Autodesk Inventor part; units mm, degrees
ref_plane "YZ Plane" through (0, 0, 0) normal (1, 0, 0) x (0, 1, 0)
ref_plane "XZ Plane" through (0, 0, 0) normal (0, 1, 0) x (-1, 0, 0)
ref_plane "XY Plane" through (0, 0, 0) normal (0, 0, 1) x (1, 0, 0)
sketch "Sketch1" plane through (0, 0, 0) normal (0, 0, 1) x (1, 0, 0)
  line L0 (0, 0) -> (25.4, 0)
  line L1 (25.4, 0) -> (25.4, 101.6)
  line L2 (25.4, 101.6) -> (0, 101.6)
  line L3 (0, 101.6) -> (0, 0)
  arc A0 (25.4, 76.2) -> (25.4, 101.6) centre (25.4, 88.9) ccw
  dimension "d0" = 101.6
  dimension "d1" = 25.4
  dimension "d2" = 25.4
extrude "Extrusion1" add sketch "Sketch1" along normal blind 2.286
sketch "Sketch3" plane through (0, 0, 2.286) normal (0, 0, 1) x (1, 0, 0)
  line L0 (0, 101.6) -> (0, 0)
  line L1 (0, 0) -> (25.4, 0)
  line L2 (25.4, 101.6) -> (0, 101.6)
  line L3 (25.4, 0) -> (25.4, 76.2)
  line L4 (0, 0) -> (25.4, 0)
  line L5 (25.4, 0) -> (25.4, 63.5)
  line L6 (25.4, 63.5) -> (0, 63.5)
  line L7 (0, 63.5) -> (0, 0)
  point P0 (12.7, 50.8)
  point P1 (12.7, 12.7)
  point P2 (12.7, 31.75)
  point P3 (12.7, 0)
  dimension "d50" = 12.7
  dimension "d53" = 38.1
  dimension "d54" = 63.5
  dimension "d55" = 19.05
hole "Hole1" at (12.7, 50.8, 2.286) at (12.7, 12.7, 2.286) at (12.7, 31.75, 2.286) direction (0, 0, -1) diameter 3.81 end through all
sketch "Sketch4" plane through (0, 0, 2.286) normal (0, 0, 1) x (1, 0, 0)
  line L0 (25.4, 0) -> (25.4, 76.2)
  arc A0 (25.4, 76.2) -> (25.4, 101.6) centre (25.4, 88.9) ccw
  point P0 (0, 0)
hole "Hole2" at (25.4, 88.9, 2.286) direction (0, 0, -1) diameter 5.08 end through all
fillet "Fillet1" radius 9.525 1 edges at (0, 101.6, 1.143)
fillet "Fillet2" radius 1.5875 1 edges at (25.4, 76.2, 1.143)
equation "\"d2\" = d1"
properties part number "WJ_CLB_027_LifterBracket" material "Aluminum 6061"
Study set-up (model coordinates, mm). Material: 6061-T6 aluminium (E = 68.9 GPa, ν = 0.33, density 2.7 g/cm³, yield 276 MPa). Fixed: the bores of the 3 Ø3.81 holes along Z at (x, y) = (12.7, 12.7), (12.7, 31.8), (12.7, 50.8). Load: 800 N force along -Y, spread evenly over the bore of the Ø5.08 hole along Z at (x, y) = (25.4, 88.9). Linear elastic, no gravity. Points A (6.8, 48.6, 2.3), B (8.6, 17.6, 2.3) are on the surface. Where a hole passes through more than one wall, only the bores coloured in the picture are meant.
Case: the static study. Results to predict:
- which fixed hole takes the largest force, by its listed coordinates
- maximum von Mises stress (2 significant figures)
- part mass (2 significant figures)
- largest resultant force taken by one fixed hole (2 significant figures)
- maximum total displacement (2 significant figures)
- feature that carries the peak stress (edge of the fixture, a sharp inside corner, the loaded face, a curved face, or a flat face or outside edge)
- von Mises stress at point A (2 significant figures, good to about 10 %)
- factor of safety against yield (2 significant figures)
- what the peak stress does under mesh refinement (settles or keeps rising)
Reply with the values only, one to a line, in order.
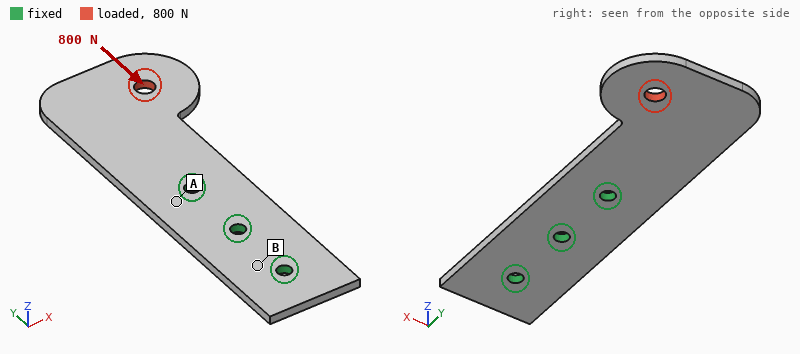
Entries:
(12.7, 50.8)
130 MPa
17 g
700 N
96 µm
a curved face
13 MPa
2.1
settles
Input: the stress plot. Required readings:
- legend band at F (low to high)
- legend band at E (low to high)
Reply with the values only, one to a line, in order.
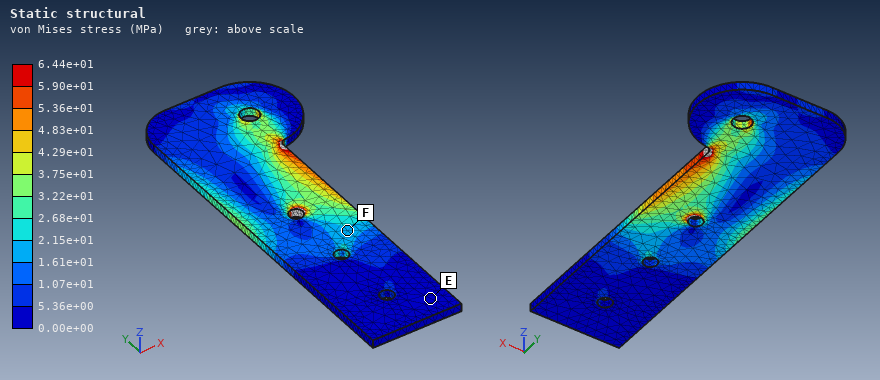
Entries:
1.61e+01 to 2.15e+01 MPa
0.00e+00 to 5.36e+00 MPa
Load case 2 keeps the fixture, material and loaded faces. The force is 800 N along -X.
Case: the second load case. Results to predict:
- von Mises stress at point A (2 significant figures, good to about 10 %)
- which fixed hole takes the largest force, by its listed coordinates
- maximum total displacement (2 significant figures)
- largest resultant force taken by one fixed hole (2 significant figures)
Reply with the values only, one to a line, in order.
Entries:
63 MPa
(12.7, 50.8)
0.23 mm
1.8 kN
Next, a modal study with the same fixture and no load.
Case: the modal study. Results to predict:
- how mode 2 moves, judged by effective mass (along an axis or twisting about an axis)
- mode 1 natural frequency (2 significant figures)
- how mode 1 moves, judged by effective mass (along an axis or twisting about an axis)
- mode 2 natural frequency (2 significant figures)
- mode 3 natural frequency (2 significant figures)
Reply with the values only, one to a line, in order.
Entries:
twisting about Y
640 Hz
along Z
1800 Hz
4200 Hz
